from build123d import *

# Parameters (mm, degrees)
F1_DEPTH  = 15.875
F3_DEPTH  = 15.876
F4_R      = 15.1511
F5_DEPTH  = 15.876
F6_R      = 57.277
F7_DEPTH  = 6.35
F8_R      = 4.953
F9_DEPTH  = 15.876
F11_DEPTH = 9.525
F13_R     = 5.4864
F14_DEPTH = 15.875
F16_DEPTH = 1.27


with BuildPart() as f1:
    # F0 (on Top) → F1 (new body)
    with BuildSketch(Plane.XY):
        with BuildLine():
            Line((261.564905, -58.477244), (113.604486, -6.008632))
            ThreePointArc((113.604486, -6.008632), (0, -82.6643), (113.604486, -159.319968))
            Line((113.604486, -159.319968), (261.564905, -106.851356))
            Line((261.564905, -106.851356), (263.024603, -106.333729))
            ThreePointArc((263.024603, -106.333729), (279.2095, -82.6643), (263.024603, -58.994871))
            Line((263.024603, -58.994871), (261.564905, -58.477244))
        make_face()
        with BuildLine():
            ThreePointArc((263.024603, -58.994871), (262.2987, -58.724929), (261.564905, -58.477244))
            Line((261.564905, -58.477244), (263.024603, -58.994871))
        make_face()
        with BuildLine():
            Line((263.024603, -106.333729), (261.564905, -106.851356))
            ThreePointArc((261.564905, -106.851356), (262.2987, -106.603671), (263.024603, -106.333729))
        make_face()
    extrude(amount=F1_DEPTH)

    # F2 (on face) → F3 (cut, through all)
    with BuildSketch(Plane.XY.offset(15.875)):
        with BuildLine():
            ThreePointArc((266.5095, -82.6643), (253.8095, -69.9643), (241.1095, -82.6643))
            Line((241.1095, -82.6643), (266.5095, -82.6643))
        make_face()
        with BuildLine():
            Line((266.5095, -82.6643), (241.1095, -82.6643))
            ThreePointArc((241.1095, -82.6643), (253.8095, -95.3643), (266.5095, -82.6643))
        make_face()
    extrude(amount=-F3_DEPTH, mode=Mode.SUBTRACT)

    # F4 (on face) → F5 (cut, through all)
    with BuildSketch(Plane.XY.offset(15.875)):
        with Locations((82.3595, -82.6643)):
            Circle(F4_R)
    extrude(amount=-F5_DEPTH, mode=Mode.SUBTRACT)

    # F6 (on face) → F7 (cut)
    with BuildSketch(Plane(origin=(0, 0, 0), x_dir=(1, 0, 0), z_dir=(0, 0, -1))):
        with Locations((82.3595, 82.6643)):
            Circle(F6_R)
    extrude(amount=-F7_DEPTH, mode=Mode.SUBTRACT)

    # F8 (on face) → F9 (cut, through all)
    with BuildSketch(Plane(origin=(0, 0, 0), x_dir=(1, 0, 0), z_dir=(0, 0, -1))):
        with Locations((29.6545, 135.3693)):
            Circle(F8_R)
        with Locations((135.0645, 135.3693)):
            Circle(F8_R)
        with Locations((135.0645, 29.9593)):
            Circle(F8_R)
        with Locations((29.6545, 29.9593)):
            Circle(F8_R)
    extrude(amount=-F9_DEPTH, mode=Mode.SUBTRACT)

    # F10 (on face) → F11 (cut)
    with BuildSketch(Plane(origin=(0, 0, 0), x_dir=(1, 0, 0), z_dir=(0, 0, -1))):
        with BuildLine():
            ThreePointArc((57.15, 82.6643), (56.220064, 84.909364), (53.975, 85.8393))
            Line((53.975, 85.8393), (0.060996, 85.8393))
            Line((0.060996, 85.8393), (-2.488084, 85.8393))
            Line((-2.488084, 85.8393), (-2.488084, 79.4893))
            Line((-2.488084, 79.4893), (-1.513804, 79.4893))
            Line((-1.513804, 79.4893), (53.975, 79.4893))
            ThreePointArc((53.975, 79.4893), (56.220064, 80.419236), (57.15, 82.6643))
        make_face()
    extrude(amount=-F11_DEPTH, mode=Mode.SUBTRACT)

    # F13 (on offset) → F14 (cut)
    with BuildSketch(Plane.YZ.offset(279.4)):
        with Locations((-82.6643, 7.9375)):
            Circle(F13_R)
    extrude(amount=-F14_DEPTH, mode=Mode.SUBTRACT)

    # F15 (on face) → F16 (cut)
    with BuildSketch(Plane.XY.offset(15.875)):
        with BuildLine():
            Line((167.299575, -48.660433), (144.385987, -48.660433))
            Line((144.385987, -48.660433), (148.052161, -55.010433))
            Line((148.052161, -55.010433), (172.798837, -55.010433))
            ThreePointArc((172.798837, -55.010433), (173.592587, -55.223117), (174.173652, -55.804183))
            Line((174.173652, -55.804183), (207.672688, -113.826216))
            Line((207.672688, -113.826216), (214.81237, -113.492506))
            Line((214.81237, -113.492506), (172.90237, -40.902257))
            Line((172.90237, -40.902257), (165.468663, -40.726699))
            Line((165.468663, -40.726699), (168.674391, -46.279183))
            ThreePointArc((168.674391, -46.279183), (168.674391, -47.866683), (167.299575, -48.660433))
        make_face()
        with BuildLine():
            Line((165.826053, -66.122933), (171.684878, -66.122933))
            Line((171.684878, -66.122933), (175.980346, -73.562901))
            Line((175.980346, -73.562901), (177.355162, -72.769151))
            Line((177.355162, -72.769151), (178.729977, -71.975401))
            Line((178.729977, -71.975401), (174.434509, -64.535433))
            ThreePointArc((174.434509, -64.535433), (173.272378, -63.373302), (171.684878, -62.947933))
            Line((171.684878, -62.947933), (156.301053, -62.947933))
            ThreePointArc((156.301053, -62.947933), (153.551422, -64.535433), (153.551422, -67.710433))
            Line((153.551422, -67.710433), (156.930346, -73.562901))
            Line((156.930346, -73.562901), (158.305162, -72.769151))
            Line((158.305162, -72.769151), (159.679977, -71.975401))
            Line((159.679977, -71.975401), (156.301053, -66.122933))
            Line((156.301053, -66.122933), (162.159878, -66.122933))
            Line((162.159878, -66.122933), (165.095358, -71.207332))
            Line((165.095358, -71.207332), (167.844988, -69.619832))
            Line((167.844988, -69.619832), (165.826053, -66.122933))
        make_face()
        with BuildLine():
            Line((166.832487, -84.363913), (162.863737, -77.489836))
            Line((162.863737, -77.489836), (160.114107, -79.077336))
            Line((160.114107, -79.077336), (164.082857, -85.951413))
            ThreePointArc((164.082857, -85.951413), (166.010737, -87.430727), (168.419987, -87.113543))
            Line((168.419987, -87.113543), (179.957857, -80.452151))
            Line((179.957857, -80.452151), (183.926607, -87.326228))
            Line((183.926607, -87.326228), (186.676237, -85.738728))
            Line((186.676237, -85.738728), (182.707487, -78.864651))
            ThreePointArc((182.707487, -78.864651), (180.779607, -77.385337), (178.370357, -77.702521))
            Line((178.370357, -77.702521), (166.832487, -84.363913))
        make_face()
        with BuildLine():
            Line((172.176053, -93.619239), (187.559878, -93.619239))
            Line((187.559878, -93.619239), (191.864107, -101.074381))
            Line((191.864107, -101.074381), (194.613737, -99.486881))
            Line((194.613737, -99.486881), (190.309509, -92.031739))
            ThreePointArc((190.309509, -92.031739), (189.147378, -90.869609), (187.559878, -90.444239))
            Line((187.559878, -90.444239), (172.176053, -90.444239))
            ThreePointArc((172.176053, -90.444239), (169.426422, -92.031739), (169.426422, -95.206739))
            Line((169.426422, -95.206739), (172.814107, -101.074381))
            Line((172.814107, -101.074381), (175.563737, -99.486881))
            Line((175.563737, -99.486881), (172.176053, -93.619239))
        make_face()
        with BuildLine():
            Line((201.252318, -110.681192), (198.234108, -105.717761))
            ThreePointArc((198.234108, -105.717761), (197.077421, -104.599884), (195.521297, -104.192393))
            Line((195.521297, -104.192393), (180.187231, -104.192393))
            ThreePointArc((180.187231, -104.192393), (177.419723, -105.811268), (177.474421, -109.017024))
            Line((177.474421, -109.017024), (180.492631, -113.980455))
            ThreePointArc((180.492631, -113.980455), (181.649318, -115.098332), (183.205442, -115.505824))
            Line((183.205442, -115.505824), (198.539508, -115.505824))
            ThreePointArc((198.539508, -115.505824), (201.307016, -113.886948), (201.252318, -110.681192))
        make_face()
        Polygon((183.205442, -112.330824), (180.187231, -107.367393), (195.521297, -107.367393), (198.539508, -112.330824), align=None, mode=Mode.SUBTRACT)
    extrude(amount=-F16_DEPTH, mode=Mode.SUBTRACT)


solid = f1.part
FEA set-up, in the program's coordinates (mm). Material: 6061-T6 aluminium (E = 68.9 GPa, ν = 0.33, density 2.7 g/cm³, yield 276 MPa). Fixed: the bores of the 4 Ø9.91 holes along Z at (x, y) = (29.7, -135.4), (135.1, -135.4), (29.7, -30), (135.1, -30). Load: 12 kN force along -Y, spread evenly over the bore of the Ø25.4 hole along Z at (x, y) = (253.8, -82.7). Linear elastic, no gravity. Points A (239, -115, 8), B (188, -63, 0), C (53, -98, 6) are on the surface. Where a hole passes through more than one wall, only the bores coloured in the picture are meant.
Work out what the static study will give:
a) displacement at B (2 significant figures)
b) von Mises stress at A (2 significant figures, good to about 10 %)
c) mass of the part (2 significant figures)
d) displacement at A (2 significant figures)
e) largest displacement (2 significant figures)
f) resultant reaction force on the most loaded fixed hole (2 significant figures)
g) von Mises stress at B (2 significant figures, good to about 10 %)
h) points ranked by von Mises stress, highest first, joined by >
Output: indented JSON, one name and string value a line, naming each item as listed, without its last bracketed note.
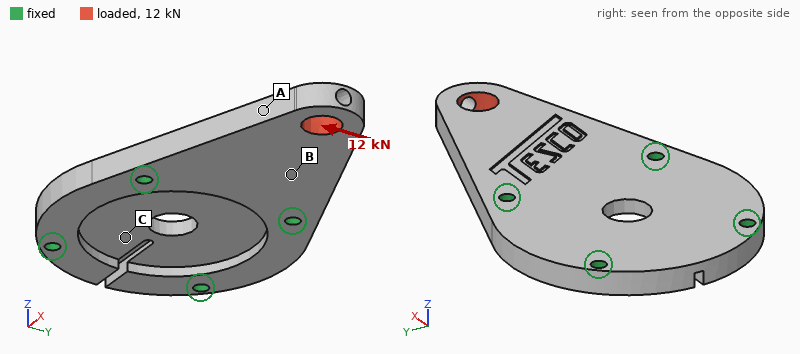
{
  "displacement at B": "0.024 mm",
  "von Mises stress at A": "35 MPa",
  "mass of the part": "1.1 kg",
  "displacement at A": "0.080 mm",
  "largest displacement": "0.13 mm",
  "resultant reaction force on the most loaded fixed hole": "14 kN",
  "von Mises stress at B": "15 MPa",
  "points ranked by von Mises stress, highest first, joined by >": "A > B > C"
}
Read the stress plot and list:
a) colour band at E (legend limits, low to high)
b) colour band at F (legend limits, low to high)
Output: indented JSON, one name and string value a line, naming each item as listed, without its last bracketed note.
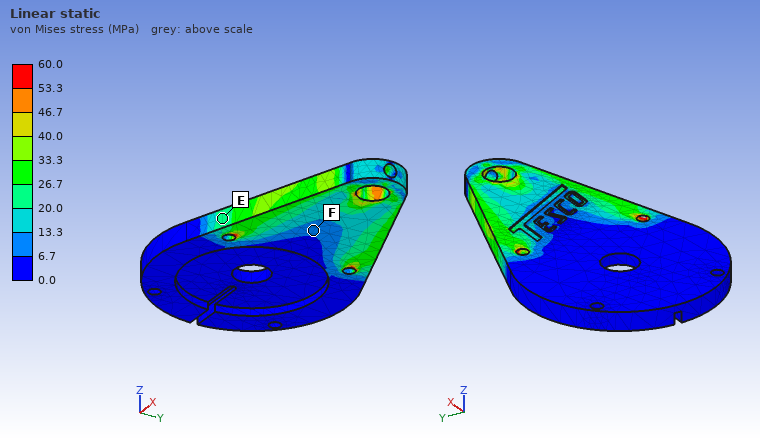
{
  "colour band at E": "20.0 to 26.7 MPa",
  "colour band at F": "6.7 to 13.3 MPa"
}
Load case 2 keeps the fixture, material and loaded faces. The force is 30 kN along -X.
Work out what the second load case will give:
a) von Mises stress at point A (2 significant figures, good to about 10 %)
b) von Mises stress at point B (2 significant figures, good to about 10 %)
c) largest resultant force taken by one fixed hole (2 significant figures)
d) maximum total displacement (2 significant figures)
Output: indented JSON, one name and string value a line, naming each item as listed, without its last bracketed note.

{
  "von Mises stress at point A": "27 MPa",
  "von Mises stress at point B": "18 MPa",
  "largest resultant force taken by one fixed hole": "14 kN",
  "maximum total displacement": "70 µm"
}
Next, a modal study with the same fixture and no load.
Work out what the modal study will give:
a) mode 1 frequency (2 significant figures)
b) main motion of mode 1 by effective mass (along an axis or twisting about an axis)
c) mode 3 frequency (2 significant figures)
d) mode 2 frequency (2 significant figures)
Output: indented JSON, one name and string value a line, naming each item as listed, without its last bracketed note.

{
  "mode 1 frequency": "850 Hz",
  "main motion of mode 1 by effective mass": "along Z",
  "mode 3 frequency": "3800 Hz",
  "mode 2 frequency": "3400 Hz"
}
